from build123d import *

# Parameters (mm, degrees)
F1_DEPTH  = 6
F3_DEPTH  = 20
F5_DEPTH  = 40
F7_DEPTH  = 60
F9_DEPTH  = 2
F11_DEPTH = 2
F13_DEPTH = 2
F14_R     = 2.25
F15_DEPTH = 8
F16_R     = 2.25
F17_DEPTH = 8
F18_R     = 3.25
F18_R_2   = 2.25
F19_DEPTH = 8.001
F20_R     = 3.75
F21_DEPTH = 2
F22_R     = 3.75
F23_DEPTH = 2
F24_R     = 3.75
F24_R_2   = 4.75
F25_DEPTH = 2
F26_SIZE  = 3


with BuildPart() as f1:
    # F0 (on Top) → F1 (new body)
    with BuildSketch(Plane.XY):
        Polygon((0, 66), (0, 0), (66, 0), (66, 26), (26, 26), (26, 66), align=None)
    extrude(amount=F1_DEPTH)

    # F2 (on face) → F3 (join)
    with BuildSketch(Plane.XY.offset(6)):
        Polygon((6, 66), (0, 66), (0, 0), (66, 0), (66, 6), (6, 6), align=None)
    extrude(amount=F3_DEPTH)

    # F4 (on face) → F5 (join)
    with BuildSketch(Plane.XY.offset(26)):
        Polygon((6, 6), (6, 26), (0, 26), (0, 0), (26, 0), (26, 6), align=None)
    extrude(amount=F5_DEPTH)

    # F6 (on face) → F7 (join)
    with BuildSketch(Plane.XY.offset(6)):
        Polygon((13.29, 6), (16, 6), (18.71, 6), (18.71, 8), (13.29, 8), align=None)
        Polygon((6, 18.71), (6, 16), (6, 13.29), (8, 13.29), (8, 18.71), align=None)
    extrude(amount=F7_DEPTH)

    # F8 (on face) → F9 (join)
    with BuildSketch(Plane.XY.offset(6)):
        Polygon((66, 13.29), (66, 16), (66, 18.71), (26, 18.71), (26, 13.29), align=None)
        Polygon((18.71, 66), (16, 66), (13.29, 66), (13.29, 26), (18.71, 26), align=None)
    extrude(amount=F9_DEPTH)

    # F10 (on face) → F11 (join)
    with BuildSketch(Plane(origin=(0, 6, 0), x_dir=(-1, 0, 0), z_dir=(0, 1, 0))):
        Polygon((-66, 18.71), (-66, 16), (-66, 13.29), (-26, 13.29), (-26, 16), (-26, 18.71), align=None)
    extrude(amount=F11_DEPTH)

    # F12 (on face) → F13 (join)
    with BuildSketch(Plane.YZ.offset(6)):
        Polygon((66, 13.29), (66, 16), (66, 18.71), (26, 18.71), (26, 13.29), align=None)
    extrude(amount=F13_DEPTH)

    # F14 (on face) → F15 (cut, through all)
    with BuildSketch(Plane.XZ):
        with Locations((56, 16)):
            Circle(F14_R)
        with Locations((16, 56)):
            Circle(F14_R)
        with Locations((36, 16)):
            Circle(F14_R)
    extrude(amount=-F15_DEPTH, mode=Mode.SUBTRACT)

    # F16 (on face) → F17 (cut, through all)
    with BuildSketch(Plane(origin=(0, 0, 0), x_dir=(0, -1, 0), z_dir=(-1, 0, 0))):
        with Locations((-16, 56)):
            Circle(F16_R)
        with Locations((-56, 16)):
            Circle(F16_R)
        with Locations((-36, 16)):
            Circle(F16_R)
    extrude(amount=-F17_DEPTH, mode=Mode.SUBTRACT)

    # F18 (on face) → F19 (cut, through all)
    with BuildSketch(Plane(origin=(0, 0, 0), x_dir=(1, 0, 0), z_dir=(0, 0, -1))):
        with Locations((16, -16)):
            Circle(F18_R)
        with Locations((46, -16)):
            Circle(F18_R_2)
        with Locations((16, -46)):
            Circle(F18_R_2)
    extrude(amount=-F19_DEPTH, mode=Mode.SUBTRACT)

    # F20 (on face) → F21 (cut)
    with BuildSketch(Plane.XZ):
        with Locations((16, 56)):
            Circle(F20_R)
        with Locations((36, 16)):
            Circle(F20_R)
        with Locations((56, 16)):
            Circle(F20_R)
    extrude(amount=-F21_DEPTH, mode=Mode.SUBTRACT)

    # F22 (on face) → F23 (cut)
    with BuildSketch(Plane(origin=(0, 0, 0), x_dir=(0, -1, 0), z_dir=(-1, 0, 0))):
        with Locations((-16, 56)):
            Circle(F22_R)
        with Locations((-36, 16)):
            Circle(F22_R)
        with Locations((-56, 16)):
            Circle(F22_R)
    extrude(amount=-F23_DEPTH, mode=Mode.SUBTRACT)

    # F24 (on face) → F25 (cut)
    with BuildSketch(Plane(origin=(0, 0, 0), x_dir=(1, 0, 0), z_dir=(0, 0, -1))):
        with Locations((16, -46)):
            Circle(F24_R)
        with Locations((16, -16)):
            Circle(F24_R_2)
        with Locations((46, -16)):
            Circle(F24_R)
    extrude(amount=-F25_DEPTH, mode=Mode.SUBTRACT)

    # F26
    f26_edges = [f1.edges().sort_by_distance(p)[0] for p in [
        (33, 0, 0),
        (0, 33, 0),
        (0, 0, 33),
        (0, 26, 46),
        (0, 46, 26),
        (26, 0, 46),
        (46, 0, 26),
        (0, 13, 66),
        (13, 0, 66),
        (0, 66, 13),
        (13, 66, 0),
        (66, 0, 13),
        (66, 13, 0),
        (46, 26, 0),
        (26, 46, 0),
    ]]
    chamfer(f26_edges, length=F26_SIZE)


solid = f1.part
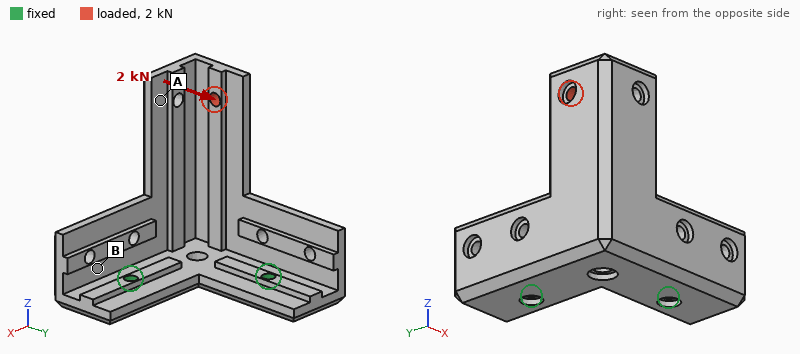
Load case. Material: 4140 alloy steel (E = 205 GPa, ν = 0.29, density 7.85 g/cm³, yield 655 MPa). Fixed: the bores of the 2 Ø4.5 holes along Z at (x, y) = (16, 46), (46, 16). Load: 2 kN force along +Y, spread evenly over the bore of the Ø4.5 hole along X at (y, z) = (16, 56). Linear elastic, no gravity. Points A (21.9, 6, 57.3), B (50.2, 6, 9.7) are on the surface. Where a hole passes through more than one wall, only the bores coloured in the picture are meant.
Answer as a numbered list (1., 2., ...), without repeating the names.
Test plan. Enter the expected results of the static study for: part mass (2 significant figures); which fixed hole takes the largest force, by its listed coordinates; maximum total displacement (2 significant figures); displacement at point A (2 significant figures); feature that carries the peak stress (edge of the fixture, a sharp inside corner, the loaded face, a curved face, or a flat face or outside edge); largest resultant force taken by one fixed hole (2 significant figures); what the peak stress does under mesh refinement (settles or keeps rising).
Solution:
1. 330 g
2. (16, 46)
3. 0.39 mm
4. 0.31 mm
5. edge of the fixture
6. 2.4 kN
7. keeps rising
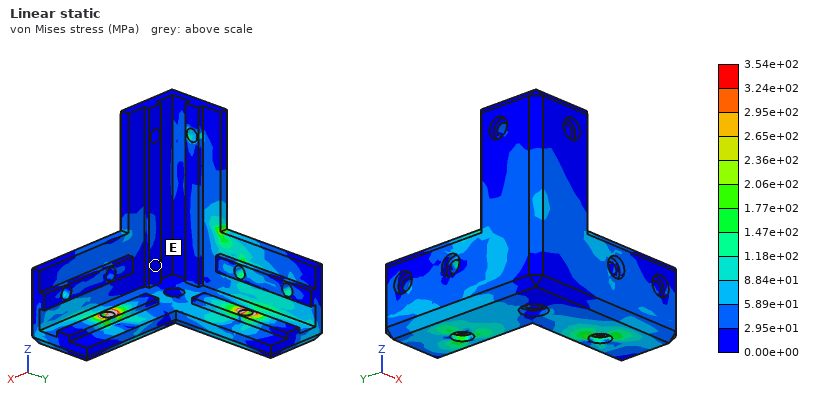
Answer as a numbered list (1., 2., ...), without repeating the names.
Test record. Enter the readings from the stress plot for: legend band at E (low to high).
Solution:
1. 0.00e+00 to 2.95e+01 MPa
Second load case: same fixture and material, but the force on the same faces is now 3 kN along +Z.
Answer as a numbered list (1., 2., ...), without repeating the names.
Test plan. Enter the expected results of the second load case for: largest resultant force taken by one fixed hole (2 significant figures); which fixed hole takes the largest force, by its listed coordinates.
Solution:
1. 1.9 kN
2. (16, 46)
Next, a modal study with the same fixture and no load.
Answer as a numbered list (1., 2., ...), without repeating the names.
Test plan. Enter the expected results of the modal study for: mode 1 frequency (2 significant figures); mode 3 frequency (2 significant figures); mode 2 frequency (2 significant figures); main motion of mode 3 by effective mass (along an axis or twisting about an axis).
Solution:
1. 1200 Hz
2. 4600 Hz
3. 2800 Hz
4. along Z
